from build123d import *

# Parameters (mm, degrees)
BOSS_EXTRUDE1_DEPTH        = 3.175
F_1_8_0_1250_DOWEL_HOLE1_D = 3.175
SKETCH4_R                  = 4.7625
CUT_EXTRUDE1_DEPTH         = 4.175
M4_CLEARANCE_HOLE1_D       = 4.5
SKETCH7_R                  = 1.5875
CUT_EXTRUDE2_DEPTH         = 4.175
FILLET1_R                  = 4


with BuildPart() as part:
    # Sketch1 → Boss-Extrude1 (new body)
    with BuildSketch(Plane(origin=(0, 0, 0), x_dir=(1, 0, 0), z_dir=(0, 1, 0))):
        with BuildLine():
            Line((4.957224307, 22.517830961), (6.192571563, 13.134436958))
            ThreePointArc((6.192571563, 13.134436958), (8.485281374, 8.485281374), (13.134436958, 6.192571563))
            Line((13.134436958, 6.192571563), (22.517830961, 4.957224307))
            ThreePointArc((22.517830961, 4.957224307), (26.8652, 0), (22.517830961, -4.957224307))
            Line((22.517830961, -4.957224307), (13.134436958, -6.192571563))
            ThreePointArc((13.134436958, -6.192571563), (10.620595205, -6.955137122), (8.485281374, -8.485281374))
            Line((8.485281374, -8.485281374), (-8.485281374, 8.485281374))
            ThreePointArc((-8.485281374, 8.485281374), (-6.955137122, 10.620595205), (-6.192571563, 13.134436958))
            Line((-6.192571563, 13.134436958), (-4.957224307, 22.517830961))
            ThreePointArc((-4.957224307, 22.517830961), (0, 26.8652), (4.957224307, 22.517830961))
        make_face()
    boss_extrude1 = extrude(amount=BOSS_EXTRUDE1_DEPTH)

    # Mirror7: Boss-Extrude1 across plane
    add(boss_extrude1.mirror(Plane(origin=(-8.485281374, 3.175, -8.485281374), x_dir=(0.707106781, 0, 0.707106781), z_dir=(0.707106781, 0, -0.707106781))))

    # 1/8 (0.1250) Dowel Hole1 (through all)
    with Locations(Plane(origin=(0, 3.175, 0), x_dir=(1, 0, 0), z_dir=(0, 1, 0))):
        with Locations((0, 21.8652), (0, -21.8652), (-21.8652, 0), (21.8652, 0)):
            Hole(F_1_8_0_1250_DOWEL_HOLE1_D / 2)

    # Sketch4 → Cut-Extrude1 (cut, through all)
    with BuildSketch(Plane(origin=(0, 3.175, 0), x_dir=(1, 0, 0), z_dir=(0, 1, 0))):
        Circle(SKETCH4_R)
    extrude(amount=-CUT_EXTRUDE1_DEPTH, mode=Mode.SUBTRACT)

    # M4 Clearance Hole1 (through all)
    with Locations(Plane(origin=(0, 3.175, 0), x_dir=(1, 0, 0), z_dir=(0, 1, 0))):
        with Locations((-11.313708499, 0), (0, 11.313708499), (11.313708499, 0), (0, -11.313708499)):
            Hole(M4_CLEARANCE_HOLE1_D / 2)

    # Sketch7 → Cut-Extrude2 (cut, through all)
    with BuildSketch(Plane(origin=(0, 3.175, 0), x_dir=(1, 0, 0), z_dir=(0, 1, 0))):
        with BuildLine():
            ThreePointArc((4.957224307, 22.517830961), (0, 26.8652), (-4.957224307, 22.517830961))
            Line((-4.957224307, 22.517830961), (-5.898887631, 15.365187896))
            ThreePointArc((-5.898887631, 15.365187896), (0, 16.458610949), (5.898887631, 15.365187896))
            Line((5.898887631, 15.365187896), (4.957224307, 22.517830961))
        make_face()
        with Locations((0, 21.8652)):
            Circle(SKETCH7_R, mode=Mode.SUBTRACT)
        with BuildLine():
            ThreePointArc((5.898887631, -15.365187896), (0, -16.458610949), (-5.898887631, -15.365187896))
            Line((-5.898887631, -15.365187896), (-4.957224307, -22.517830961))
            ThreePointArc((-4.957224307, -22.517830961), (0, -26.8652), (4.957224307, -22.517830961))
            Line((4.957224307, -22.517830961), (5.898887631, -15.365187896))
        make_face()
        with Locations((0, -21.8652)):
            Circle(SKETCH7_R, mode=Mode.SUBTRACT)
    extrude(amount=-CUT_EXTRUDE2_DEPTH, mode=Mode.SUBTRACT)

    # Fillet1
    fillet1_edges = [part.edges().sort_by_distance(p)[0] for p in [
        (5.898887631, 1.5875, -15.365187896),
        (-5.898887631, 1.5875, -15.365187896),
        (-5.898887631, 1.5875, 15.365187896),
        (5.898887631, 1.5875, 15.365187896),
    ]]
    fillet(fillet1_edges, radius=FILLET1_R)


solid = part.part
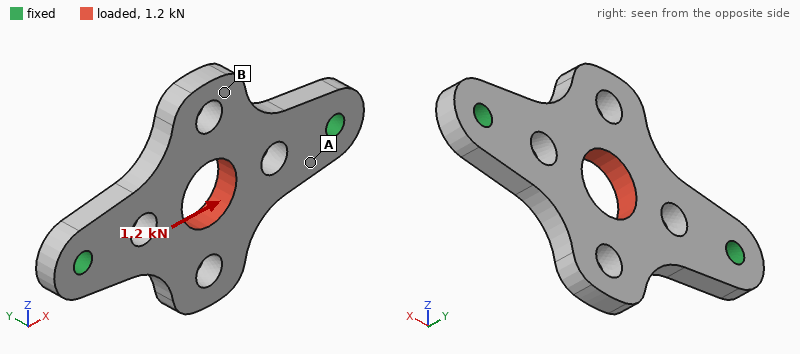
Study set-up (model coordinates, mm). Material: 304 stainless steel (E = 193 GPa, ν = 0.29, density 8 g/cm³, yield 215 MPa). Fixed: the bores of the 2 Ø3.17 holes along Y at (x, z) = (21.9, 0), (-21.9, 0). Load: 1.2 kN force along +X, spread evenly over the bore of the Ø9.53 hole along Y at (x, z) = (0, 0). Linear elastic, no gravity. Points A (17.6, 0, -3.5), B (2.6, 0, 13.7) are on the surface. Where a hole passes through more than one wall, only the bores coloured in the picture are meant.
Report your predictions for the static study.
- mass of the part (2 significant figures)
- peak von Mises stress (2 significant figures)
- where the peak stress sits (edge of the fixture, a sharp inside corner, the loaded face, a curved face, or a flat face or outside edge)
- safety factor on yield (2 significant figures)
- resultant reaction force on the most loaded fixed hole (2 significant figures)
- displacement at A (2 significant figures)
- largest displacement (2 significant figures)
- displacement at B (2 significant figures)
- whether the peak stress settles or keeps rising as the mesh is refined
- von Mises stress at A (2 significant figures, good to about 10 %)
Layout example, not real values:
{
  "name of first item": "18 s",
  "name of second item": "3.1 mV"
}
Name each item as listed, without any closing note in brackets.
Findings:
{
  "mass of the part": "19 g",
  "peak von Mises stress": "52 MPa",
  "where the peak stress sits": "a curved face",
  "safety factor on yield": "4.1",
  "resultant reaction force on the most loaded fixed hole": "600 N",
  "displacement at A": "0.56 µm",
  "largest displacement": "2.1 µm",
  "displacement at B": "1.4 µm",
  "whether the peak stress settles or keeps rising as the mesh is refined": "settles",
  "von Mises stress at A": "19 MPa"
}
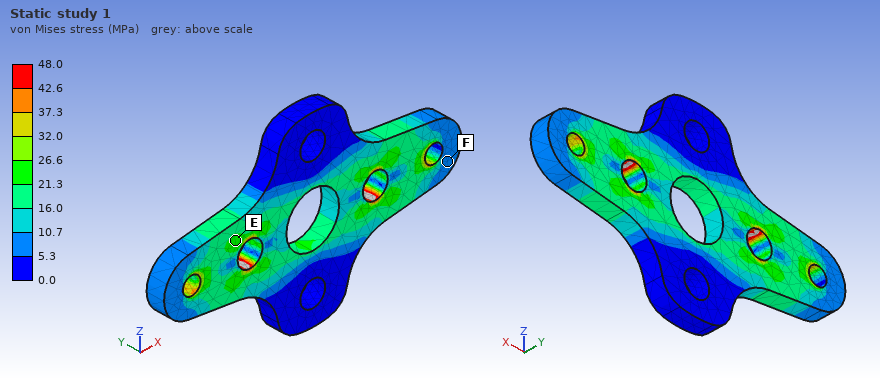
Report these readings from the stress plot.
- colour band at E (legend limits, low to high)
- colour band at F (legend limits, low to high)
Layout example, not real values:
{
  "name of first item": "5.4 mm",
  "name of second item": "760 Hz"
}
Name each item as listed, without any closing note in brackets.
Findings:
{
  "colour band at E": "21.3 to 26.6 MPa",
  "colour band at F": "5.3 to 10.7 MPa"
}
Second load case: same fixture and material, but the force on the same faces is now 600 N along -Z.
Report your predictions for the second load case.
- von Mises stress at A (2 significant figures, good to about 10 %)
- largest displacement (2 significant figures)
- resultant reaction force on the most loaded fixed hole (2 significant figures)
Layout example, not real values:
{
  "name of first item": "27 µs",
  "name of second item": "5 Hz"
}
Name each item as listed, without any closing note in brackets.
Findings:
{
  "von Mises stress at A": "12 MPa",
  "largest displacement": "4.5 µm",
  "resultant reaction force on the most loaded fixed hole": "300 N"
}
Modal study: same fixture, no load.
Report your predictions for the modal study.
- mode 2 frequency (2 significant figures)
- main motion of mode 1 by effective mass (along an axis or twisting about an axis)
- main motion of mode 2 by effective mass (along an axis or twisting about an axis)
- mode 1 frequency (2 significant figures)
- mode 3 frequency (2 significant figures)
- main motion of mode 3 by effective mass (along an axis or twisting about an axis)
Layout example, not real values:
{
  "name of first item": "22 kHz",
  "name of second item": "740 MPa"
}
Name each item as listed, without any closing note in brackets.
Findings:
{
  "mode 2 frequency": "6000 Hz",
  "main motion of mode 1 by effective mass": "twisting about X",
  "main motion of mode 2 by effective mass": "along Y",
  "mode 1 frequency": "5400 Hz",
  "mode 3 frequency": "18 kHz",
  "main motion of mode 3 by effective mass": "along Z"
}
